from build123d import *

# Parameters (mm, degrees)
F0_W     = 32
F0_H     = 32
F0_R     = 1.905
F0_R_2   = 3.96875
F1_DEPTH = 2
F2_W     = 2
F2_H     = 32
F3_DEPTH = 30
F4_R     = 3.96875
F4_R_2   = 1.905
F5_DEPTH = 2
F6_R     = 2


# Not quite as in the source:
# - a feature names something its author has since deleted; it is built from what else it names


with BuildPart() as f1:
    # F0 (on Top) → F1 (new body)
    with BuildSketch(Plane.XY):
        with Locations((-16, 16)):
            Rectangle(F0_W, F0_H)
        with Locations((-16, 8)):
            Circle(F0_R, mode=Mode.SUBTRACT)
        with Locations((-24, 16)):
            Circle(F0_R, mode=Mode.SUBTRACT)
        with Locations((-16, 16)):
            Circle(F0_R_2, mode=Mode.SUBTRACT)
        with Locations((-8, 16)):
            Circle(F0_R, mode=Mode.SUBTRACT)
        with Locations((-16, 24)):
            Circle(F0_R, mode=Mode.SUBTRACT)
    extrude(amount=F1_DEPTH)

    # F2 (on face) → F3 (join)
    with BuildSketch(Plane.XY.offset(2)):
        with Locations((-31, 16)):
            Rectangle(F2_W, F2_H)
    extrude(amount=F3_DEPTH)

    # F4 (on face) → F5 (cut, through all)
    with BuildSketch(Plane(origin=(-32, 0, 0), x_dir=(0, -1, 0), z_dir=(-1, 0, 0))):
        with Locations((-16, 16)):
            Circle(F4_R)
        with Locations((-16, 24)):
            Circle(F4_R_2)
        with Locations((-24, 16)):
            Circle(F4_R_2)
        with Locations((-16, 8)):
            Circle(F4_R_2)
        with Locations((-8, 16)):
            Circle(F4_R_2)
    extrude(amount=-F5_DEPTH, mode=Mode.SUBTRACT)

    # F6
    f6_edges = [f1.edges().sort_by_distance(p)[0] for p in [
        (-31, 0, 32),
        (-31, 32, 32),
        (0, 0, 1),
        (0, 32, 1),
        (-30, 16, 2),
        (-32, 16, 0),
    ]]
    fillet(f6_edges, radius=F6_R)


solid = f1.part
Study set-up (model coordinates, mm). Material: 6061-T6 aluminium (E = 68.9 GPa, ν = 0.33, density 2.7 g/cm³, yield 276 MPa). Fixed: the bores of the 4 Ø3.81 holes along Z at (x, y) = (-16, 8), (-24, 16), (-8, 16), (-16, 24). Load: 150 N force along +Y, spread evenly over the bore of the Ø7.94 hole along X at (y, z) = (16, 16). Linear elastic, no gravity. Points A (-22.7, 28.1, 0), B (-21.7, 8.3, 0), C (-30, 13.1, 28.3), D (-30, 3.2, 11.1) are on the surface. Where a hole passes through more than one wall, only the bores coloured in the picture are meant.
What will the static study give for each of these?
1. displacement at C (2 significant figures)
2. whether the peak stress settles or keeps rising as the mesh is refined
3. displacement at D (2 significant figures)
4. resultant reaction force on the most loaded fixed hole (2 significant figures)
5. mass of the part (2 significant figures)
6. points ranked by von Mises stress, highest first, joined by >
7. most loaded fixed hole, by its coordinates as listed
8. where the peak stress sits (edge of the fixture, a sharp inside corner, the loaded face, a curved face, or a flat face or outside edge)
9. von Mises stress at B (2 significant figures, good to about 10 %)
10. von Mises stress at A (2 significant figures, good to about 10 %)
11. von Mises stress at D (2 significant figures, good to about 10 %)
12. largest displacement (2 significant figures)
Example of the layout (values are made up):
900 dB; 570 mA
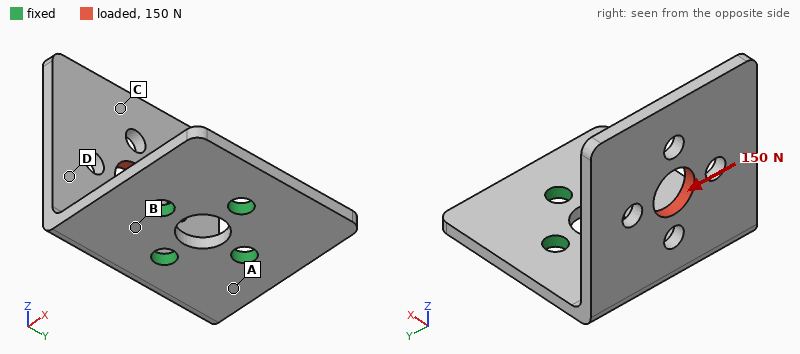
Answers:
0.12 mm; keeps rising; 0.072 mm; 130 N; 9.7 g; B > A > D > C; (-24, 16); edge of the fixture; 41 MPa; 29 MPa; 16 MPa; 0.15 mm
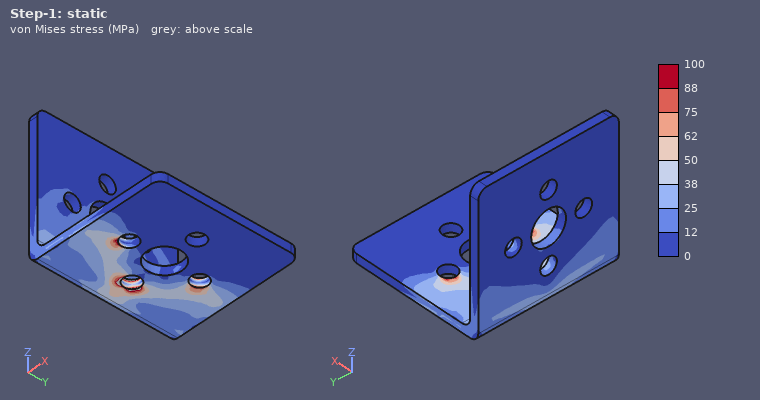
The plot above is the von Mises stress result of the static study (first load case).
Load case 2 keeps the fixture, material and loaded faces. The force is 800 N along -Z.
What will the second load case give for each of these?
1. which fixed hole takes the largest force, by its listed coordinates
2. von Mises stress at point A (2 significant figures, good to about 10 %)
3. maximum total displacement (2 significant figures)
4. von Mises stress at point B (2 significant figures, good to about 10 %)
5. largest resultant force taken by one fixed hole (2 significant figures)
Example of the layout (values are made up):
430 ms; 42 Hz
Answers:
(-24, 16); 60 MPa; 0.42 mm; 62 MPa; 940 N
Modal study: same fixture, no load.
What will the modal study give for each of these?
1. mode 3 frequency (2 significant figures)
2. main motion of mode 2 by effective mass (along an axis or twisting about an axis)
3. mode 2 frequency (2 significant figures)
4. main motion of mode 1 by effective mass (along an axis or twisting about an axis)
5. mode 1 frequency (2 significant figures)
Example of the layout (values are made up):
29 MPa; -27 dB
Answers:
3800 Hz; along Y; 2400 Hz; along X; 1400 Hz
